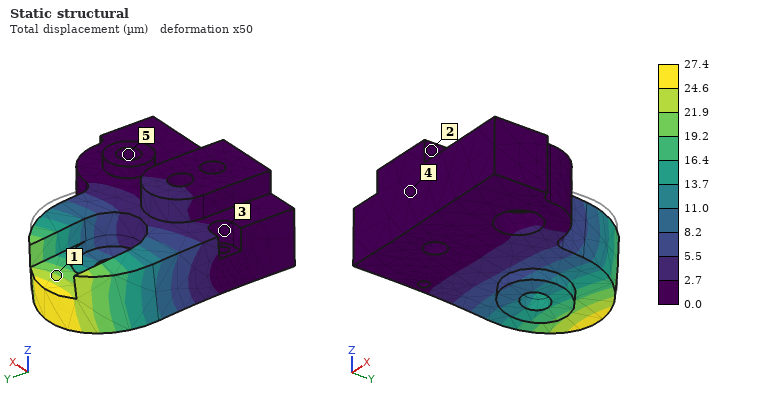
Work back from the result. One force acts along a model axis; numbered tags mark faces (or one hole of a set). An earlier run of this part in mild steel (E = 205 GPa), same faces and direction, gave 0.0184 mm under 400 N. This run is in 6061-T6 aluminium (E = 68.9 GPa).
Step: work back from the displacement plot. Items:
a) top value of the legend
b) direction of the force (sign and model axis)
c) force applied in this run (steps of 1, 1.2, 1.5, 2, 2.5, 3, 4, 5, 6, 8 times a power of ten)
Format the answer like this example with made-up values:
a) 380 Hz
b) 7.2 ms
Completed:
a) 27.4 µm
b) -Z
c) 200 N
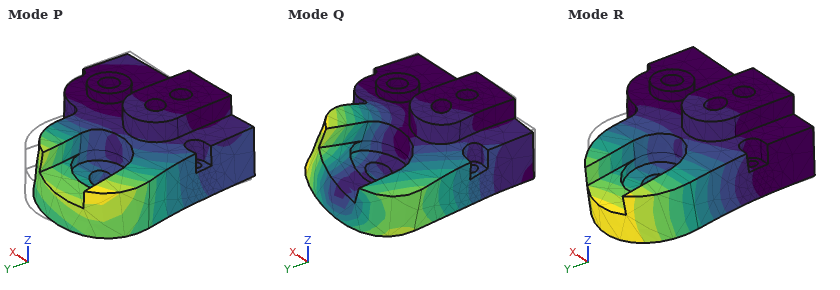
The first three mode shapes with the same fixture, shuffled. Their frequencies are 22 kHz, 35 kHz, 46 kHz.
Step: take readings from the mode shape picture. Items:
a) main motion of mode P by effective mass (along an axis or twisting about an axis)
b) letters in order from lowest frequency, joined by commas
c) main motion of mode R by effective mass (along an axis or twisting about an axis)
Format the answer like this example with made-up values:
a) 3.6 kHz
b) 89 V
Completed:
a) along X
b) R, P, Q
c) along Z
